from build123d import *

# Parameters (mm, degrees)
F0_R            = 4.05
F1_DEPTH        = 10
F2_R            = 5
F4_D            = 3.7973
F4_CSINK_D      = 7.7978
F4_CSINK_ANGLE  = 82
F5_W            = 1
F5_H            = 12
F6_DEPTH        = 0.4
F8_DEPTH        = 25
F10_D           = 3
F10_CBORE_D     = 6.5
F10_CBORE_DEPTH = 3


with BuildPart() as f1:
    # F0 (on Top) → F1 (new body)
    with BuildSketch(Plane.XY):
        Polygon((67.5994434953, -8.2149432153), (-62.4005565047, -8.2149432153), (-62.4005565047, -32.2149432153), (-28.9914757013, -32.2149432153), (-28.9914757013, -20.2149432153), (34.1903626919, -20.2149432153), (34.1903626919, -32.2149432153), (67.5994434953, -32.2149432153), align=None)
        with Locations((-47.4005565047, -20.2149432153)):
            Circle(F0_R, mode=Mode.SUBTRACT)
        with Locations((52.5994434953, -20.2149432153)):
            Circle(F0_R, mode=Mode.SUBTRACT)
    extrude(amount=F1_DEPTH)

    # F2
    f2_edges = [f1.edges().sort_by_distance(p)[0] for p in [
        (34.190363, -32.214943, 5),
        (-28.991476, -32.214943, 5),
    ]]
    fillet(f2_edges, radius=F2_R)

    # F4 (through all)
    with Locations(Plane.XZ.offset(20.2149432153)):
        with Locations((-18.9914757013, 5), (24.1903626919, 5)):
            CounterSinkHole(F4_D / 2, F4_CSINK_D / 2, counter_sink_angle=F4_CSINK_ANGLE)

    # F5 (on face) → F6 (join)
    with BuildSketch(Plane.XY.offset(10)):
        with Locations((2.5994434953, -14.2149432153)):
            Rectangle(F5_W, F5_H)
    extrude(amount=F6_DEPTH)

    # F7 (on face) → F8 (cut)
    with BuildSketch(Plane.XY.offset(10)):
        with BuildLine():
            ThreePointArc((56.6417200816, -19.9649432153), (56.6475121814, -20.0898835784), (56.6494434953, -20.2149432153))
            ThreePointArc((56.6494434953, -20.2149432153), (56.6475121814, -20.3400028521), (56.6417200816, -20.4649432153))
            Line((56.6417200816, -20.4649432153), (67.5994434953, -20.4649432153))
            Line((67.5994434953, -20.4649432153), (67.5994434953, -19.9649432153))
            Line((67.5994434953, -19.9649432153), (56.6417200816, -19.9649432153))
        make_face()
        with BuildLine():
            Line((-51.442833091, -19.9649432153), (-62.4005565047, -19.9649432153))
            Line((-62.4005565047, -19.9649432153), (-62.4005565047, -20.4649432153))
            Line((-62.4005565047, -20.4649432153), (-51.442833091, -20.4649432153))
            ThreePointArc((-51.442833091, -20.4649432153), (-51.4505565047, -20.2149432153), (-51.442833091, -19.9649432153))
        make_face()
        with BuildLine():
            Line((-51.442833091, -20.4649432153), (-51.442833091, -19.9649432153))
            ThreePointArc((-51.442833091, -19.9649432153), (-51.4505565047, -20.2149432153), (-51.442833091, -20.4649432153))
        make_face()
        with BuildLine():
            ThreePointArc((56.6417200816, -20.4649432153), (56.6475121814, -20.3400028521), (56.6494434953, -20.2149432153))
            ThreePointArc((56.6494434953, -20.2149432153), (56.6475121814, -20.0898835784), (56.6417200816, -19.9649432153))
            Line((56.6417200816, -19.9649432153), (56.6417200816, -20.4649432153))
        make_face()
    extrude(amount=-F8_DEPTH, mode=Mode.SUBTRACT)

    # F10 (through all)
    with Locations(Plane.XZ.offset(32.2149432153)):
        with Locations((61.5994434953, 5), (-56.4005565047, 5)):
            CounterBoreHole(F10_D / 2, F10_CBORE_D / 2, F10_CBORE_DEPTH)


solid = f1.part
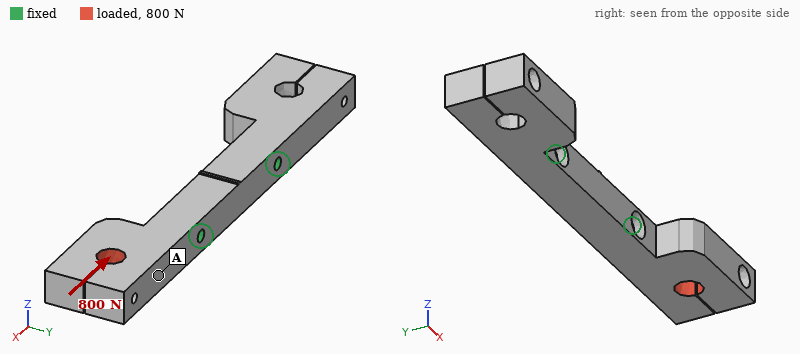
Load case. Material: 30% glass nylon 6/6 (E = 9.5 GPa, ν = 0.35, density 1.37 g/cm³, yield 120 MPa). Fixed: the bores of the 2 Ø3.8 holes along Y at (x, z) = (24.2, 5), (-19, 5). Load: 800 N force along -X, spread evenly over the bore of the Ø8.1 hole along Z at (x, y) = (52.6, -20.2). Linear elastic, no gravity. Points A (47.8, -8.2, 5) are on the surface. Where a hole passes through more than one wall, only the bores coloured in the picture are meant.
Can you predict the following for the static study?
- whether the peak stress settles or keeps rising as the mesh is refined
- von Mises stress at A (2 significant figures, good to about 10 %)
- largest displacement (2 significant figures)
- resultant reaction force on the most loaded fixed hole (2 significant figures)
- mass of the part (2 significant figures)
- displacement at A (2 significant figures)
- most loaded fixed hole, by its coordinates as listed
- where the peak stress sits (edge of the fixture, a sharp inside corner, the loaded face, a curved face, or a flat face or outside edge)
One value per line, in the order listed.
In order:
keeps rising
4.7 MPa
0.27 mm
760 N
30 g
0.10 mm
(24.2, 5)
edge of the fixture
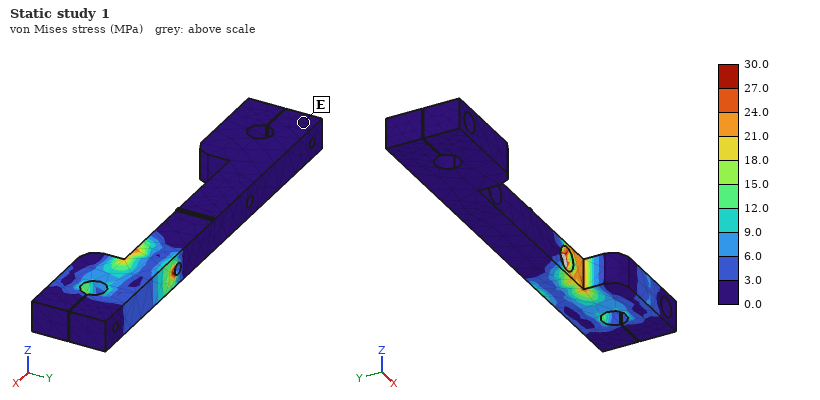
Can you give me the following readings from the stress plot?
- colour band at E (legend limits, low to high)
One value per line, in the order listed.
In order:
0.0 to 3.0 MPa
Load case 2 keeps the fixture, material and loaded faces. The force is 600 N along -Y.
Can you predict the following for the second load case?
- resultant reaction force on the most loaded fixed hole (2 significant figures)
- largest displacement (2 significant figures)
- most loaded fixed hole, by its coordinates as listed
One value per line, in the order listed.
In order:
650 N
0.75 mm
(24.2, 5)
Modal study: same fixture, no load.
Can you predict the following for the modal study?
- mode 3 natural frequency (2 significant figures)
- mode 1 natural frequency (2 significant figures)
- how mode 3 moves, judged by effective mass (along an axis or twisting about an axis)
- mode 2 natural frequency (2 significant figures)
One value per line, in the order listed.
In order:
1800 Hz
1500 Hz
along Y
1500 Hz
